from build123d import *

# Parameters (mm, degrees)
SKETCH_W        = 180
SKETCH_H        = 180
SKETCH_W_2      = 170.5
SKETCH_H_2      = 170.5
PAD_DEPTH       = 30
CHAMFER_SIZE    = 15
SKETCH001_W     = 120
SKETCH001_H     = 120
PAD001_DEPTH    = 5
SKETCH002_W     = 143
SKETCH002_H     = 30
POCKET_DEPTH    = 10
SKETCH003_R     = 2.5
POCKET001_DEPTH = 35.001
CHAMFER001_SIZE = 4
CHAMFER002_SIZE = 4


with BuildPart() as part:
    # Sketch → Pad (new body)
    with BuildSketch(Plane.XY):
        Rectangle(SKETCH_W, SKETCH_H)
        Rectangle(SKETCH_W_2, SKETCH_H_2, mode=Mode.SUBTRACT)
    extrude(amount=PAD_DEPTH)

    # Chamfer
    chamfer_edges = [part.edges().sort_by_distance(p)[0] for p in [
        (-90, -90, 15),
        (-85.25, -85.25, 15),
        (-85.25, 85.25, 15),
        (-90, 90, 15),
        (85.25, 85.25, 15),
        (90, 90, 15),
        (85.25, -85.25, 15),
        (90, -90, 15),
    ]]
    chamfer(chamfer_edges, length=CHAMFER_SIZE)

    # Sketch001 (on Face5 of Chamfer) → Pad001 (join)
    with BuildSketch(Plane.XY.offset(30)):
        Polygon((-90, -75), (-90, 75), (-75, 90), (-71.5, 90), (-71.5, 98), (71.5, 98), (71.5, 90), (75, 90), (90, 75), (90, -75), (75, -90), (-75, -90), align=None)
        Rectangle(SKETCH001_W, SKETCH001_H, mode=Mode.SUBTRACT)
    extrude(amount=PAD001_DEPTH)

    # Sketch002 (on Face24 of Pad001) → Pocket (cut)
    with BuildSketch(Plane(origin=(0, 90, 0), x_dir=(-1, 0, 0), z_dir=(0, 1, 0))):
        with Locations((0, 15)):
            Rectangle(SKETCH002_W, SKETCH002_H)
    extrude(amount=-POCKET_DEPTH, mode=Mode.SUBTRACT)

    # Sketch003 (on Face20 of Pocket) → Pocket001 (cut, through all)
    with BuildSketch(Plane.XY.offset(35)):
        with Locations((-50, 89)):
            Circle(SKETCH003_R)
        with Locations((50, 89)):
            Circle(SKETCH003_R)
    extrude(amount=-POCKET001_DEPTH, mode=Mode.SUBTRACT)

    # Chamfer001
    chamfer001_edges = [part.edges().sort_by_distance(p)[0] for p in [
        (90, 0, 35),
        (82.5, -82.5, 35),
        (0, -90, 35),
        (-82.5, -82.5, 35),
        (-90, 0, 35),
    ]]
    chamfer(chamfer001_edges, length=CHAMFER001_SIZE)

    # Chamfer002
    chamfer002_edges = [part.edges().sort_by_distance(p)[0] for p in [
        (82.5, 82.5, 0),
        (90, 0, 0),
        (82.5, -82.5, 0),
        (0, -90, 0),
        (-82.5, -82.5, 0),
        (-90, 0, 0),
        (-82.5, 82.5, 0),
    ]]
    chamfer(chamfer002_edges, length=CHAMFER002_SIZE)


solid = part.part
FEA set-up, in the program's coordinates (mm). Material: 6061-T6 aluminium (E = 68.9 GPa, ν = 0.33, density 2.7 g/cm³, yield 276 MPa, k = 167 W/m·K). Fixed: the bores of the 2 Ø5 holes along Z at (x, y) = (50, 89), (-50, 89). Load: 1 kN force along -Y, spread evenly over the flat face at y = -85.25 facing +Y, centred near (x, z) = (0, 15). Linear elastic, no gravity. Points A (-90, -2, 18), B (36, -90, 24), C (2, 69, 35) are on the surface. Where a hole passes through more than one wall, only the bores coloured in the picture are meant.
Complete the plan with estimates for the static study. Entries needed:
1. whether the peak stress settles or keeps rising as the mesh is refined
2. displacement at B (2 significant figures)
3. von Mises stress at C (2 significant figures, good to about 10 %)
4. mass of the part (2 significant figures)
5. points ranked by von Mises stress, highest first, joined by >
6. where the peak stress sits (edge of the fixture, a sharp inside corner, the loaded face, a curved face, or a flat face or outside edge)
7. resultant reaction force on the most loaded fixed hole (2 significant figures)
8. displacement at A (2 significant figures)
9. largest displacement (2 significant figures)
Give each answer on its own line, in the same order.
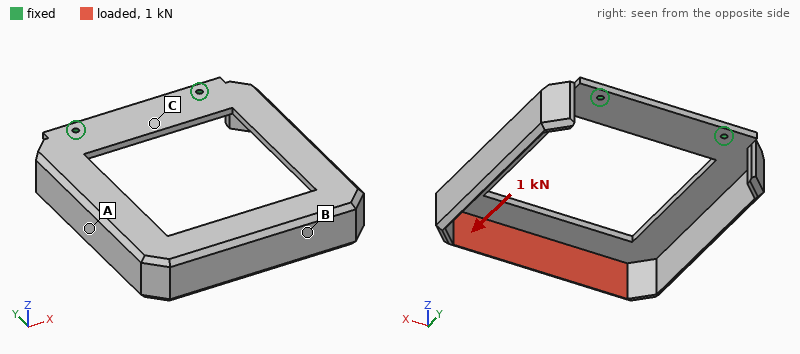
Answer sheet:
keeps rising
1.2 mm
10 MPa
440 g
B > C > A
edge of the fixture
710 N
0.58 mm
1.3 mm
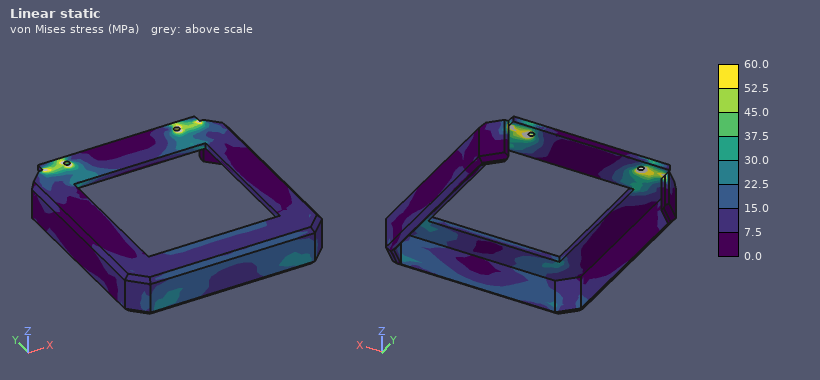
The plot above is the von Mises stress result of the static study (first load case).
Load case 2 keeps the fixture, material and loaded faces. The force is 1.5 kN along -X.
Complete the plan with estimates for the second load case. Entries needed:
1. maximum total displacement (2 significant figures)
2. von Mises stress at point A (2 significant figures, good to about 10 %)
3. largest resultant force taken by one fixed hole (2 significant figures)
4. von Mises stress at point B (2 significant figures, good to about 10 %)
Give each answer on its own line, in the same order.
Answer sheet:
2.2 mm
22 MPa
2.5 kN
31 MPa
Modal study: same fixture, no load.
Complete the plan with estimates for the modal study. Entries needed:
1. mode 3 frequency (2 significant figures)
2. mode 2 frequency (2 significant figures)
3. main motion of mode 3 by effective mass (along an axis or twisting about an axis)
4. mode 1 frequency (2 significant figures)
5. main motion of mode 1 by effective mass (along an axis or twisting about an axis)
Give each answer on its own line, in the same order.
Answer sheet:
560 Hz
200 Hz
along X
110 Hz
along Z
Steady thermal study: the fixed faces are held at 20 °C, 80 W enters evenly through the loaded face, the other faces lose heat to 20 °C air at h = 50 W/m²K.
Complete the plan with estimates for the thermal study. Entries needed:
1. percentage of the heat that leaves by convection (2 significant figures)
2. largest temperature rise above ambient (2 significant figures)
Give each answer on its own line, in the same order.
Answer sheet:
90 %
63 K
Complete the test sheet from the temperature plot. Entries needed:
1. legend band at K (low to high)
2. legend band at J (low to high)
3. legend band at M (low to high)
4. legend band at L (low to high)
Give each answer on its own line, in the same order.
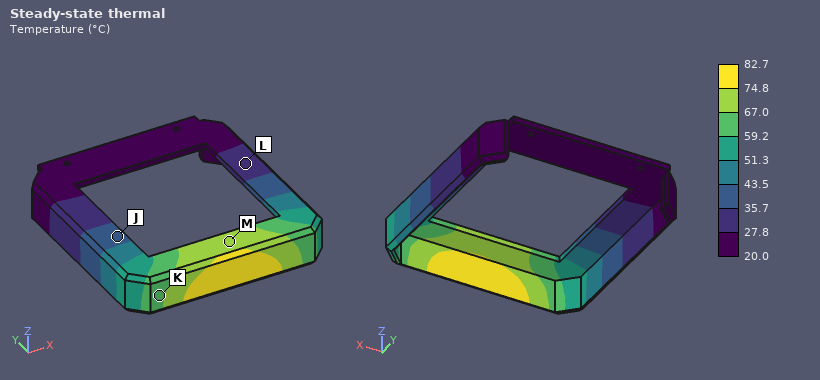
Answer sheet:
59.2 to 67.0 °C
35.7 to 43.5 °C
67.0 to 74.8 °C
27.8 to 35.7 °C
